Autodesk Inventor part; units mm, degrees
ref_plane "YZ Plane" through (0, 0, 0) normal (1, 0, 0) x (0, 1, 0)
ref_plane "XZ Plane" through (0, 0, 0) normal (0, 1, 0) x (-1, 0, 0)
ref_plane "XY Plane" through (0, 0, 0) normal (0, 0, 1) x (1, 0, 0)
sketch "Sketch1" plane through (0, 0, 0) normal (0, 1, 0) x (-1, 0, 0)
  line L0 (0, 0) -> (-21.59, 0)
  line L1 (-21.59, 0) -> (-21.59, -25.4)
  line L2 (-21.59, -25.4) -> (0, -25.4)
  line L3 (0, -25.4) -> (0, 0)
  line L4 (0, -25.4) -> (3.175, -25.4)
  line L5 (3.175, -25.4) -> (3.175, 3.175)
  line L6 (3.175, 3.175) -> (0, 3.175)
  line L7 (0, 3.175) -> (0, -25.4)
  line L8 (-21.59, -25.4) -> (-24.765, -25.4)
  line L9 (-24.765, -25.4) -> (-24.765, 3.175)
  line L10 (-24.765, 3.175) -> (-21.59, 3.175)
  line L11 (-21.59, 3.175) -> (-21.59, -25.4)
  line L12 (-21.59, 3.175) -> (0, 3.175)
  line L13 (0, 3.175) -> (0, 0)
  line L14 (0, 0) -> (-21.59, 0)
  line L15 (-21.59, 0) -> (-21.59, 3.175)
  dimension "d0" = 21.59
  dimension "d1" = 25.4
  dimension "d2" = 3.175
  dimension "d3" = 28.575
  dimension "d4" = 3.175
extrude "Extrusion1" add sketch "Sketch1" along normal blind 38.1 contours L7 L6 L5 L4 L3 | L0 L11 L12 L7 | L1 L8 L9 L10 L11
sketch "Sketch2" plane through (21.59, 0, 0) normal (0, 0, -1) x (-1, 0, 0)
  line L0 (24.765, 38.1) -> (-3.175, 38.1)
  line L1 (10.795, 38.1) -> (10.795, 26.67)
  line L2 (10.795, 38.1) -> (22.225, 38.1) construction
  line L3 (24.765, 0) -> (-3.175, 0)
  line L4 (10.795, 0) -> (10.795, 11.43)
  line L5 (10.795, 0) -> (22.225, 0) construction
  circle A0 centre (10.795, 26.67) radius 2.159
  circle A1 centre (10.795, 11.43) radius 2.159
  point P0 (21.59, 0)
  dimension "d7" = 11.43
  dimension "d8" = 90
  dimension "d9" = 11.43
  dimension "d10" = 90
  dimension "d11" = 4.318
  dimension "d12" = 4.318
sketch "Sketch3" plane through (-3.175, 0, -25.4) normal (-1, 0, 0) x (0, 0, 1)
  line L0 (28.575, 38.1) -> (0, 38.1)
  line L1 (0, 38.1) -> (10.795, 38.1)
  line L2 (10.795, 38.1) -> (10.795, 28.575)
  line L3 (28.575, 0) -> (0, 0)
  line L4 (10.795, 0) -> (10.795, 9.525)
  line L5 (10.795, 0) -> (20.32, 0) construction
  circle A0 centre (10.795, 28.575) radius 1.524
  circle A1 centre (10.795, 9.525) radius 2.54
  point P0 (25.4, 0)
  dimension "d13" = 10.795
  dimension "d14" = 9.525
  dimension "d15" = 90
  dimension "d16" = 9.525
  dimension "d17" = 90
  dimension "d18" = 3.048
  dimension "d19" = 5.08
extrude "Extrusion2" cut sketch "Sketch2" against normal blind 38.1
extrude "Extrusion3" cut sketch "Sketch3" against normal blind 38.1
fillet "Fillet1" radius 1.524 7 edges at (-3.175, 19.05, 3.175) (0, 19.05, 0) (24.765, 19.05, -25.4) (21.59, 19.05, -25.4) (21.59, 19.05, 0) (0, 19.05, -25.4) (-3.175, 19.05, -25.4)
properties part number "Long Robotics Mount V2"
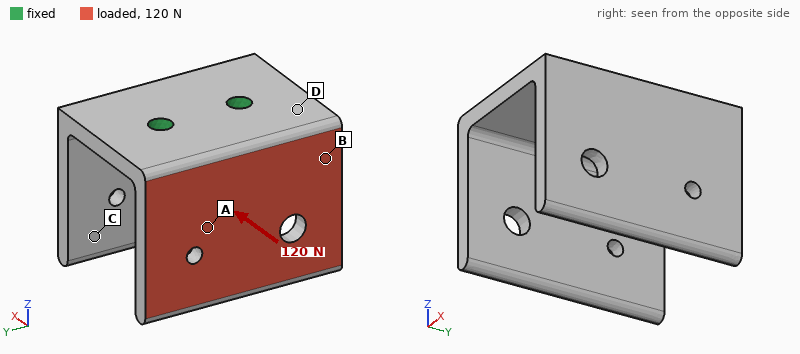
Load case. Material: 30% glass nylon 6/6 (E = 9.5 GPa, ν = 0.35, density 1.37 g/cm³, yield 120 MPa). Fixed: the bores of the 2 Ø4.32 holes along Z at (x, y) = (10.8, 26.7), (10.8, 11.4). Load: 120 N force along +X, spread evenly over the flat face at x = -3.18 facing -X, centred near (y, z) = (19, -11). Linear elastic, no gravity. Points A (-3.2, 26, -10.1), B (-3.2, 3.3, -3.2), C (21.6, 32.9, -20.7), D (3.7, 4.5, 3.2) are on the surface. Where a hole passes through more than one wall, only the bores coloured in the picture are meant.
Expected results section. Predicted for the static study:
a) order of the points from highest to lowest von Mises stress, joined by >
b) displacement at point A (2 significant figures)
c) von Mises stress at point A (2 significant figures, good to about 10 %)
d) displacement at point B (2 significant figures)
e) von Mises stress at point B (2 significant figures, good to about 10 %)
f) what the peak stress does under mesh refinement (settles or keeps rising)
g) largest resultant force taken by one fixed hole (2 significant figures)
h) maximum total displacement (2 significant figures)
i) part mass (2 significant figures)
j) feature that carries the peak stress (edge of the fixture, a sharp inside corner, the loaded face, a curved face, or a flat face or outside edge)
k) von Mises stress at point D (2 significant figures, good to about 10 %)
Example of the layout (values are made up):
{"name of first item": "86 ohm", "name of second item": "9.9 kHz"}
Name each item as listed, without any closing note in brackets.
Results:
{"order of the points from highest to lowest von Mises stress, joined by >": "D > B > A > C", "displacement at point A": "0.28 mm", "von Mises stress at point A": "6.2 MPa", "displacement at point B": "0.16 mm", "von Mises stress at point B": "14 MPa", "what the peak stress does under mesh refinement": "keeps rising", "largest resultant force taken by one fixed hole": "62 N", "maximum total displacement": "0.65 mm", "part mass": "13 g", "feature that carries the peak stress": "edge of the fixture", "von Mises stress at point D": "19 MPa"}
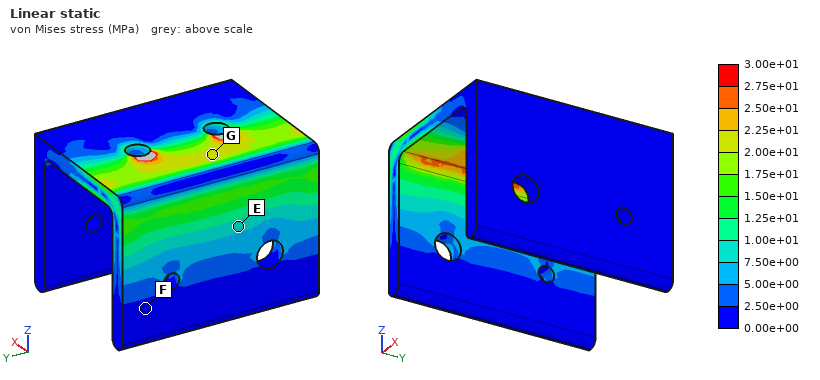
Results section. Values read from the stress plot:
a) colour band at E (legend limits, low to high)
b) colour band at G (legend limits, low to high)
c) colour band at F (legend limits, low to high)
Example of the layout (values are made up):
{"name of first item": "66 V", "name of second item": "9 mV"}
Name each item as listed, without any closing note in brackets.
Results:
{"colour band at E": "7.50e+00 to 1.00e+01 MPa", "colour band at G": "2.00e+01 to 2.25e+01 MPa", "colour band at F": "0.00e+00 to 2.50e+00 MPa"}
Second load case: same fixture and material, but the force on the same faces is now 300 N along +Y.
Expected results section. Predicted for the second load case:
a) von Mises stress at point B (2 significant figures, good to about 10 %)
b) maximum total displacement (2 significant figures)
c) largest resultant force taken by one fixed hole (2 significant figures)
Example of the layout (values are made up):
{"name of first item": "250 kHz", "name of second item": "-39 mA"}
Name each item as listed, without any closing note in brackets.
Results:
{"von Mises stress at point B": "11 MPa", "maximum total displacement": "0.34 mm", "largest resultant force taken by one fixed hole": "320 N"}
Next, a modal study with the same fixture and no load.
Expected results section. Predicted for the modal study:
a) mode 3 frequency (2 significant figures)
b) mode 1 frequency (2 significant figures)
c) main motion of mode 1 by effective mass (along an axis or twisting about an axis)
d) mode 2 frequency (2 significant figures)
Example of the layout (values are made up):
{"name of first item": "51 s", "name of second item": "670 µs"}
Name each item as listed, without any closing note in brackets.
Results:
{"mode 3 frequency": "2100 Hz", "mode 1 frequency": "1200 Hz", "main motion of mode 1 by effective mass": "along X", "mode 2 frequency": "1200 Hz"}
